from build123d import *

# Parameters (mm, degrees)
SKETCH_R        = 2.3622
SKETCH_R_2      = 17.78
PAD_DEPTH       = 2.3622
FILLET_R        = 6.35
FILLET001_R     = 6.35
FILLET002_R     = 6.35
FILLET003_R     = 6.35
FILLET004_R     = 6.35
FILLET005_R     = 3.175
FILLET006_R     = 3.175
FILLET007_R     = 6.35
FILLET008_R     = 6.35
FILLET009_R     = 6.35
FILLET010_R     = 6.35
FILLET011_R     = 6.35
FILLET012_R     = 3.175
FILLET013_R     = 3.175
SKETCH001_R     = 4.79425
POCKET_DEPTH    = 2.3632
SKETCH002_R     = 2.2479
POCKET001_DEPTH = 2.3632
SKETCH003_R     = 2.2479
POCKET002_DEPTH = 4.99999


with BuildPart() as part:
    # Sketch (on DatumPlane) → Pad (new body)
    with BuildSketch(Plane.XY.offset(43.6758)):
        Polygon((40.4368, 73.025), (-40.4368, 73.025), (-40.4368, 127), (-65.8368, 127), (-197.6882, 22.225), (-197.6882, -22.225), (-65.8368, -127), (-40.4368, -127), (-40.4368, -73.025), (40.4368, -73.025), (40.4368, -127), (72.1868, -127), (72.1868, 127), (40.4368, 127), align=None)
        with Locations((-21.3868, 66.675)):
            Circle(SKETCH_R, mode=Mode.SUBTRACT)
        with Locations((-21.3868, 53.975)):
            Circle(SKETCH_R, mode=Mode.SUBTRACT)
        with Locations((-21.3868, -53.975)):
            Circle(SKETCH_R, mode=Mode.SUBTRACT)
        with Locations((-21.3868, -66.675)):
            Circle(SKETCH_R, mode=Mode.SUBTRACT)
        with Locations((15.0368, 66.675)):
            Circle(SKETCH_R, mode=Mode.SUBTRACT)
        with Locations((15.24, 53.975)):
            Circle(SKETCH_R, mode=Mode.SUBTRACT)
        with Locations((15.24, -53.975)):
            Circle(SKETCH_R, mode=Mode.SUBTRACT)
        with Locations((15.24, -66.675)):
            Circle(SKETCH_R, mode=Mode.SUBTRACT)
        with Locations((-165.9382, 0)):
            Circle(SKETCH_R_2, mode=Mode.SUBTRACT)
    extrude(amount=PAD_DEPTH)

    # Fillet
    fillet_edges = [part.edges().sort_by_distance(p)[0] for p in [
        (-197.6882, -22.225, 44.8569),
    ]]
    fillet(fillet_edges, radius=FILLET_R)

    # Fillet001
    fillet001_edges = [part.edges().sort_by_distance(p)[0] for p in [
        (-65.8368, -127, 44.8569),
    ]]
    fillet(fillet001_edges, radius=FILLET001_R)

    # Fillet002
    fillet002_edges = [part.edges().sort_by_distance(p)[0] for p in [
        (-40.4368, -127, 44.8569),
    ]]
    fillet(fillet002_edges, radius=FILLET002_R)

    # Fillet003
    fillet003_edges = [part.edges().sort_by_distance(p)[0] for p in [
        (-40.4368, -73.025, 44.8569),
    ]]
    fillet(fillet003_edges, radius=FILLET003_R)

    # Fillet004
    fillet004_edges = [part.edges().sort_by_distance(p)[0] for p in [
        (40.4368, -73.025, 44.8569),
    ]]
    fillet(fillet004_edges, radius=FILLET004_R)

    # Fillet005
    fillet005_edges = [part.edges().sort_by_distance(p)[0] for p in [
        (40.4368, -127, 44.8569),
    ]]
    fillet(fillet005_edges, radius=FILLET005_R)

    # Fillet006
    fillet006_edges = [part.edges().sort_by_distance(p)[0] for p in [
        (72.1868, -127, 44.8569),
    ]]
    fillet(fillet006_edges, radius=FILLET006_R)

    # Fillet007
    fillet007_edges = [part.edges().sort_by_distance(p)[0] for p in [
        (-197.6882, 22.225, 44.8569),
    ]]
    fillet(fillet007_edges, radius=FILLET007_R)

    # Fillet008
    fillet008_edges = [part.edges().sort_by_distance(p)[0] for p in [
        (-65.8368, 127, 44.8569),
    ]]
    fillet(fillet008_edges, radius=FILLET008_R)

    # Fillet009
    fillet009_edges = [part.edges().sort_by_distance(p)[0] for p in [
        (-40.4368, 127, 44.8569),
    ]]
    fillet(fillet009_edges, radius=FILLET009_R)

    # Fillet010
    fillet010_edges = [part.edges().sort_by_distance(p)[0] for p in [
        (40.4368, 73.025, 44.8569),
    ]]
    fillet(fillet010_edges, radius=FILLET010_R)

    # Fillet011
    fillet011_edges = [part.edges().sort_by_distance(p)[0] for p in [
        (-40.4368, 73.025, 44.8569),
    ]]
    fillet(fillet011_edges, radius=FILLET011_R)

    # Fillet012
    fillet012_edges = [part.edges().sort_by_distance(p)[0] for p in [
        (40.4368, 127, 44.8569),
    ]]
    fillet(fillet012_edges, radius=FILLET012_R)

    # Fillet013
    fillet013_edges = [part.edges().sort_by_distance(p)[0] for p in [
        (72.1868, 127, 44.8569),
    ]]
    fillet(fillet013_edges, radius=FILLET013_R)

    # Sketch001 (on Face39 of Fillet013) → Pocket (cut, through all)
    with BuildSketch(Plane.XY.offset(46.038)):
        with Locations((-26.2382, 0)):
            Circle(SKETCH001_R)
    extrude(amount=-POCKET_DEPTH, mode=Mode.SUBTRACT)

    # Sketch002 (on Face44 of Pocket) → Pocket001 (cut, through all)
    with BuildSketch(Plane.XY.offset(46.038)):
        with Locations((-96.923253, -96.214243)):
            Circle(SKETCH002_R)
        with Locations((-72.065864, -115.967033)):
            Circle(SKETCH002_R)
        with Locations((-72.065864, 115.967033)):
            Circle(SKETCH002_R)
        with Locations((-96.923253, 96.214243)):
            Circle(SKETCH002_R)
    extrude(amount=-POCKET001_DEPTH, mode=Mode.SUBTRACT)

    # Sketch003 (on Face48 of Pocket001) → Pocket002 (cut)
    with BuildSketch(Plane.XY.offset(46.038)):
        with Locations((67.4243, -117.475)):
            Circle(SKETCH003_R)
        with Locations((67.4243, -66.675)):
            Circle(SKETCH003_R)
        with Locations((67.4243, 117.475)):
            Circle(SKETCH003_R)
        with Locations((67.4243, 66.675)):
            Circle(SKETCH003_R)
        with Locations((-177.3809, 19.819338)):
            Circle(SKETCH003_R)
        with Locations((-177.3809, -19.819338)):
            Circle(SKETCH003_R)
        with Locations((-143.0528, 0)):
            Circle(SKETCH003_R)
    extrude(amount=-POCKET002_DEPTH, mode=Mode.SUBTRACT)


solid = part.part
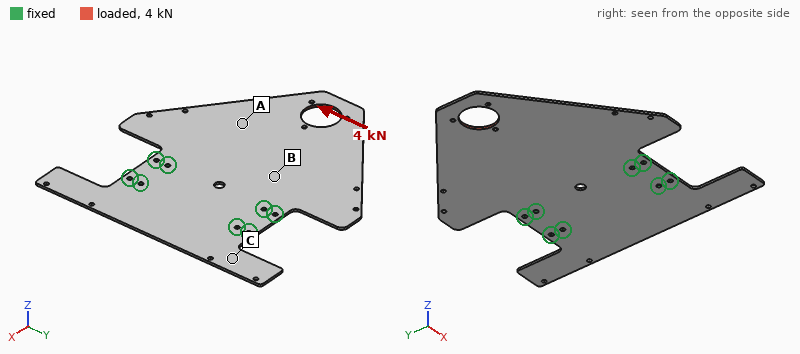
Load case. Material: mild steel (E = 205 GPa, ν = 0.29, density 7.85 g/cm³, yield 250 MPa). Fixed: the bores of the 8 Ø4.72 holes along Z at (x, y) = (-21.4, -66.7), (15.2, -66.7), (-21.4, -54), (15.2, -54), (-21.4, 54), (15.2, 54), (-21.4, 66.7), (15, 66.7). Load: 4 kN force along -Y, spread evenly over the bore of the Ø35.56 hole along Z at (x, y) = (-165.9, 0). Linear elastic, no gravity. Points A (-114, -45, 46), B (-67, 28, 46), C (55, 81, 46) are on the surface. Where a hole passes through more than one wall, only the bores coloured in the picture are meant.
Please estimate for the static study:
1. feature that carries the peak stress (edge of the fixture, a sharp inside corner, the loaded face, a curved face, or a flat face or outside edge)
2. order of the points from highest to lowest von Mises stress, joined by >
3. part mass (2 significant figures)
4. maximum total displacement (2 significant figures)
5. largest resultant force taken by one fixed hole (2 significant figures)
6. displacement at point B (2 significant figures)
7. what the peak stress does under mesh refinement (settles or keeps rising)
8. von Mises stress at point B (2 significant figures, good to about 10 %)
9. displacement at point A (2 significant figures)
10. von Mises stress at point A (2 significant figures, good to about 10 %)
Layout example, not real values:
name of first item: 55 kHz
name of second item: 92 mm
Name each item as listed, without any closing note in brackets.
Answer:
feature that carries the peak stress: edge of the fixture
order of the points from highest to lowest von Mises stress, joined by >: B > A > C
part mass: 830 g
maximum total displacement: 71 µm
largest resultant force taken by one fixed hole: 2.6 kN
displacement at point B: 14 µm
what the peak stress does under mesh refinement: keeps rising
von Mises stress at point B: 31 MPa
displacement at point A: 33 µm
von Mises stress at point A: 19 MPa
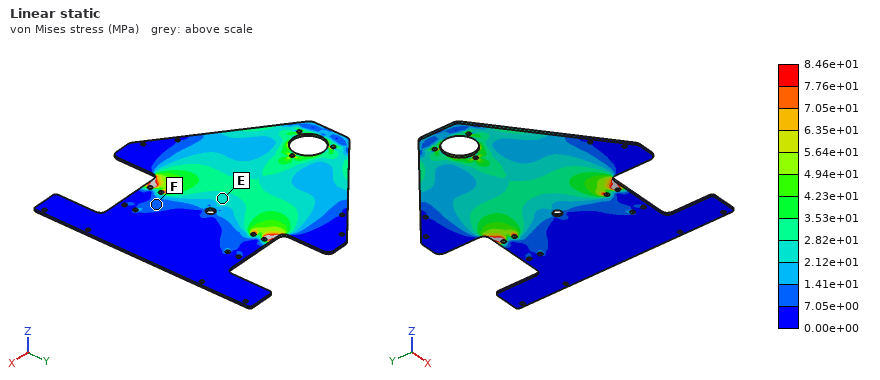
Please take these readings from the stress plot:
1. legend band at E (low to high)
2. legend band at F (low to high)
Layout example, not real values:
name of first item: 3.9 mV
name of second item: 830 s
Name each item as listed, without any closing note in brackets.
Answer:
legend band at E: 2.12e+01 to 2.82e+01 MPa
legend band at F: 7.05e+00 to 1.41e+01 MPa
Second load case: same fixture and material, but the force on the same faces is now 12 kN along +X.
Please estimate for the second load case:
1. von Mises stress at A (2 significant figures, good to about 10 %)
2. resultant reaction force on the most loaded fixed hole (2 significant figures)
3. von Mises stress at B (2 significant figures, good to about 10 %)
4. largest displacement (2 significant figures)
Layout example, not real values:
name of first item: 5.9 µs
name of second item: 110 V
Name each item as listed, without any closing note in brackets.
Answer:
von Mises stress at A: 36 MPa
resultant reaction force on the most loaded fixed hole: 2.6 kN
von Mises stress at B: 35 MPa
largest displacement: 55 µm
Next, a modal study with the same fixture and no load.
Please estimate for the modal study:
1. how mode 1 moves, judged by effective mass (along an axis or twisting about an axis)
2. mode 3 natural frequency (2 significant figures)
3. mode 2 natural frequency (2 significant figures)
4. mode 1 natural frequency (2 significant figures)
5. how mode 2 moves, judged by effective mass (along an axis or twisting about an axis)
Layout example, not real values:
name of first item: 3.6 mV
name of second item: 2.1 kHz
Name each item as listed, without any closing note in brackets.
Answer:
how mode 1 moves, judged by effective mass: along Z
mode 3 natural frequency: 310 Hz
mode 2 natural frequency: 200 Hz
mode 1 natural frequency: 83 Hz
how mode 2 moves, judged by effective mass: twisting about X
